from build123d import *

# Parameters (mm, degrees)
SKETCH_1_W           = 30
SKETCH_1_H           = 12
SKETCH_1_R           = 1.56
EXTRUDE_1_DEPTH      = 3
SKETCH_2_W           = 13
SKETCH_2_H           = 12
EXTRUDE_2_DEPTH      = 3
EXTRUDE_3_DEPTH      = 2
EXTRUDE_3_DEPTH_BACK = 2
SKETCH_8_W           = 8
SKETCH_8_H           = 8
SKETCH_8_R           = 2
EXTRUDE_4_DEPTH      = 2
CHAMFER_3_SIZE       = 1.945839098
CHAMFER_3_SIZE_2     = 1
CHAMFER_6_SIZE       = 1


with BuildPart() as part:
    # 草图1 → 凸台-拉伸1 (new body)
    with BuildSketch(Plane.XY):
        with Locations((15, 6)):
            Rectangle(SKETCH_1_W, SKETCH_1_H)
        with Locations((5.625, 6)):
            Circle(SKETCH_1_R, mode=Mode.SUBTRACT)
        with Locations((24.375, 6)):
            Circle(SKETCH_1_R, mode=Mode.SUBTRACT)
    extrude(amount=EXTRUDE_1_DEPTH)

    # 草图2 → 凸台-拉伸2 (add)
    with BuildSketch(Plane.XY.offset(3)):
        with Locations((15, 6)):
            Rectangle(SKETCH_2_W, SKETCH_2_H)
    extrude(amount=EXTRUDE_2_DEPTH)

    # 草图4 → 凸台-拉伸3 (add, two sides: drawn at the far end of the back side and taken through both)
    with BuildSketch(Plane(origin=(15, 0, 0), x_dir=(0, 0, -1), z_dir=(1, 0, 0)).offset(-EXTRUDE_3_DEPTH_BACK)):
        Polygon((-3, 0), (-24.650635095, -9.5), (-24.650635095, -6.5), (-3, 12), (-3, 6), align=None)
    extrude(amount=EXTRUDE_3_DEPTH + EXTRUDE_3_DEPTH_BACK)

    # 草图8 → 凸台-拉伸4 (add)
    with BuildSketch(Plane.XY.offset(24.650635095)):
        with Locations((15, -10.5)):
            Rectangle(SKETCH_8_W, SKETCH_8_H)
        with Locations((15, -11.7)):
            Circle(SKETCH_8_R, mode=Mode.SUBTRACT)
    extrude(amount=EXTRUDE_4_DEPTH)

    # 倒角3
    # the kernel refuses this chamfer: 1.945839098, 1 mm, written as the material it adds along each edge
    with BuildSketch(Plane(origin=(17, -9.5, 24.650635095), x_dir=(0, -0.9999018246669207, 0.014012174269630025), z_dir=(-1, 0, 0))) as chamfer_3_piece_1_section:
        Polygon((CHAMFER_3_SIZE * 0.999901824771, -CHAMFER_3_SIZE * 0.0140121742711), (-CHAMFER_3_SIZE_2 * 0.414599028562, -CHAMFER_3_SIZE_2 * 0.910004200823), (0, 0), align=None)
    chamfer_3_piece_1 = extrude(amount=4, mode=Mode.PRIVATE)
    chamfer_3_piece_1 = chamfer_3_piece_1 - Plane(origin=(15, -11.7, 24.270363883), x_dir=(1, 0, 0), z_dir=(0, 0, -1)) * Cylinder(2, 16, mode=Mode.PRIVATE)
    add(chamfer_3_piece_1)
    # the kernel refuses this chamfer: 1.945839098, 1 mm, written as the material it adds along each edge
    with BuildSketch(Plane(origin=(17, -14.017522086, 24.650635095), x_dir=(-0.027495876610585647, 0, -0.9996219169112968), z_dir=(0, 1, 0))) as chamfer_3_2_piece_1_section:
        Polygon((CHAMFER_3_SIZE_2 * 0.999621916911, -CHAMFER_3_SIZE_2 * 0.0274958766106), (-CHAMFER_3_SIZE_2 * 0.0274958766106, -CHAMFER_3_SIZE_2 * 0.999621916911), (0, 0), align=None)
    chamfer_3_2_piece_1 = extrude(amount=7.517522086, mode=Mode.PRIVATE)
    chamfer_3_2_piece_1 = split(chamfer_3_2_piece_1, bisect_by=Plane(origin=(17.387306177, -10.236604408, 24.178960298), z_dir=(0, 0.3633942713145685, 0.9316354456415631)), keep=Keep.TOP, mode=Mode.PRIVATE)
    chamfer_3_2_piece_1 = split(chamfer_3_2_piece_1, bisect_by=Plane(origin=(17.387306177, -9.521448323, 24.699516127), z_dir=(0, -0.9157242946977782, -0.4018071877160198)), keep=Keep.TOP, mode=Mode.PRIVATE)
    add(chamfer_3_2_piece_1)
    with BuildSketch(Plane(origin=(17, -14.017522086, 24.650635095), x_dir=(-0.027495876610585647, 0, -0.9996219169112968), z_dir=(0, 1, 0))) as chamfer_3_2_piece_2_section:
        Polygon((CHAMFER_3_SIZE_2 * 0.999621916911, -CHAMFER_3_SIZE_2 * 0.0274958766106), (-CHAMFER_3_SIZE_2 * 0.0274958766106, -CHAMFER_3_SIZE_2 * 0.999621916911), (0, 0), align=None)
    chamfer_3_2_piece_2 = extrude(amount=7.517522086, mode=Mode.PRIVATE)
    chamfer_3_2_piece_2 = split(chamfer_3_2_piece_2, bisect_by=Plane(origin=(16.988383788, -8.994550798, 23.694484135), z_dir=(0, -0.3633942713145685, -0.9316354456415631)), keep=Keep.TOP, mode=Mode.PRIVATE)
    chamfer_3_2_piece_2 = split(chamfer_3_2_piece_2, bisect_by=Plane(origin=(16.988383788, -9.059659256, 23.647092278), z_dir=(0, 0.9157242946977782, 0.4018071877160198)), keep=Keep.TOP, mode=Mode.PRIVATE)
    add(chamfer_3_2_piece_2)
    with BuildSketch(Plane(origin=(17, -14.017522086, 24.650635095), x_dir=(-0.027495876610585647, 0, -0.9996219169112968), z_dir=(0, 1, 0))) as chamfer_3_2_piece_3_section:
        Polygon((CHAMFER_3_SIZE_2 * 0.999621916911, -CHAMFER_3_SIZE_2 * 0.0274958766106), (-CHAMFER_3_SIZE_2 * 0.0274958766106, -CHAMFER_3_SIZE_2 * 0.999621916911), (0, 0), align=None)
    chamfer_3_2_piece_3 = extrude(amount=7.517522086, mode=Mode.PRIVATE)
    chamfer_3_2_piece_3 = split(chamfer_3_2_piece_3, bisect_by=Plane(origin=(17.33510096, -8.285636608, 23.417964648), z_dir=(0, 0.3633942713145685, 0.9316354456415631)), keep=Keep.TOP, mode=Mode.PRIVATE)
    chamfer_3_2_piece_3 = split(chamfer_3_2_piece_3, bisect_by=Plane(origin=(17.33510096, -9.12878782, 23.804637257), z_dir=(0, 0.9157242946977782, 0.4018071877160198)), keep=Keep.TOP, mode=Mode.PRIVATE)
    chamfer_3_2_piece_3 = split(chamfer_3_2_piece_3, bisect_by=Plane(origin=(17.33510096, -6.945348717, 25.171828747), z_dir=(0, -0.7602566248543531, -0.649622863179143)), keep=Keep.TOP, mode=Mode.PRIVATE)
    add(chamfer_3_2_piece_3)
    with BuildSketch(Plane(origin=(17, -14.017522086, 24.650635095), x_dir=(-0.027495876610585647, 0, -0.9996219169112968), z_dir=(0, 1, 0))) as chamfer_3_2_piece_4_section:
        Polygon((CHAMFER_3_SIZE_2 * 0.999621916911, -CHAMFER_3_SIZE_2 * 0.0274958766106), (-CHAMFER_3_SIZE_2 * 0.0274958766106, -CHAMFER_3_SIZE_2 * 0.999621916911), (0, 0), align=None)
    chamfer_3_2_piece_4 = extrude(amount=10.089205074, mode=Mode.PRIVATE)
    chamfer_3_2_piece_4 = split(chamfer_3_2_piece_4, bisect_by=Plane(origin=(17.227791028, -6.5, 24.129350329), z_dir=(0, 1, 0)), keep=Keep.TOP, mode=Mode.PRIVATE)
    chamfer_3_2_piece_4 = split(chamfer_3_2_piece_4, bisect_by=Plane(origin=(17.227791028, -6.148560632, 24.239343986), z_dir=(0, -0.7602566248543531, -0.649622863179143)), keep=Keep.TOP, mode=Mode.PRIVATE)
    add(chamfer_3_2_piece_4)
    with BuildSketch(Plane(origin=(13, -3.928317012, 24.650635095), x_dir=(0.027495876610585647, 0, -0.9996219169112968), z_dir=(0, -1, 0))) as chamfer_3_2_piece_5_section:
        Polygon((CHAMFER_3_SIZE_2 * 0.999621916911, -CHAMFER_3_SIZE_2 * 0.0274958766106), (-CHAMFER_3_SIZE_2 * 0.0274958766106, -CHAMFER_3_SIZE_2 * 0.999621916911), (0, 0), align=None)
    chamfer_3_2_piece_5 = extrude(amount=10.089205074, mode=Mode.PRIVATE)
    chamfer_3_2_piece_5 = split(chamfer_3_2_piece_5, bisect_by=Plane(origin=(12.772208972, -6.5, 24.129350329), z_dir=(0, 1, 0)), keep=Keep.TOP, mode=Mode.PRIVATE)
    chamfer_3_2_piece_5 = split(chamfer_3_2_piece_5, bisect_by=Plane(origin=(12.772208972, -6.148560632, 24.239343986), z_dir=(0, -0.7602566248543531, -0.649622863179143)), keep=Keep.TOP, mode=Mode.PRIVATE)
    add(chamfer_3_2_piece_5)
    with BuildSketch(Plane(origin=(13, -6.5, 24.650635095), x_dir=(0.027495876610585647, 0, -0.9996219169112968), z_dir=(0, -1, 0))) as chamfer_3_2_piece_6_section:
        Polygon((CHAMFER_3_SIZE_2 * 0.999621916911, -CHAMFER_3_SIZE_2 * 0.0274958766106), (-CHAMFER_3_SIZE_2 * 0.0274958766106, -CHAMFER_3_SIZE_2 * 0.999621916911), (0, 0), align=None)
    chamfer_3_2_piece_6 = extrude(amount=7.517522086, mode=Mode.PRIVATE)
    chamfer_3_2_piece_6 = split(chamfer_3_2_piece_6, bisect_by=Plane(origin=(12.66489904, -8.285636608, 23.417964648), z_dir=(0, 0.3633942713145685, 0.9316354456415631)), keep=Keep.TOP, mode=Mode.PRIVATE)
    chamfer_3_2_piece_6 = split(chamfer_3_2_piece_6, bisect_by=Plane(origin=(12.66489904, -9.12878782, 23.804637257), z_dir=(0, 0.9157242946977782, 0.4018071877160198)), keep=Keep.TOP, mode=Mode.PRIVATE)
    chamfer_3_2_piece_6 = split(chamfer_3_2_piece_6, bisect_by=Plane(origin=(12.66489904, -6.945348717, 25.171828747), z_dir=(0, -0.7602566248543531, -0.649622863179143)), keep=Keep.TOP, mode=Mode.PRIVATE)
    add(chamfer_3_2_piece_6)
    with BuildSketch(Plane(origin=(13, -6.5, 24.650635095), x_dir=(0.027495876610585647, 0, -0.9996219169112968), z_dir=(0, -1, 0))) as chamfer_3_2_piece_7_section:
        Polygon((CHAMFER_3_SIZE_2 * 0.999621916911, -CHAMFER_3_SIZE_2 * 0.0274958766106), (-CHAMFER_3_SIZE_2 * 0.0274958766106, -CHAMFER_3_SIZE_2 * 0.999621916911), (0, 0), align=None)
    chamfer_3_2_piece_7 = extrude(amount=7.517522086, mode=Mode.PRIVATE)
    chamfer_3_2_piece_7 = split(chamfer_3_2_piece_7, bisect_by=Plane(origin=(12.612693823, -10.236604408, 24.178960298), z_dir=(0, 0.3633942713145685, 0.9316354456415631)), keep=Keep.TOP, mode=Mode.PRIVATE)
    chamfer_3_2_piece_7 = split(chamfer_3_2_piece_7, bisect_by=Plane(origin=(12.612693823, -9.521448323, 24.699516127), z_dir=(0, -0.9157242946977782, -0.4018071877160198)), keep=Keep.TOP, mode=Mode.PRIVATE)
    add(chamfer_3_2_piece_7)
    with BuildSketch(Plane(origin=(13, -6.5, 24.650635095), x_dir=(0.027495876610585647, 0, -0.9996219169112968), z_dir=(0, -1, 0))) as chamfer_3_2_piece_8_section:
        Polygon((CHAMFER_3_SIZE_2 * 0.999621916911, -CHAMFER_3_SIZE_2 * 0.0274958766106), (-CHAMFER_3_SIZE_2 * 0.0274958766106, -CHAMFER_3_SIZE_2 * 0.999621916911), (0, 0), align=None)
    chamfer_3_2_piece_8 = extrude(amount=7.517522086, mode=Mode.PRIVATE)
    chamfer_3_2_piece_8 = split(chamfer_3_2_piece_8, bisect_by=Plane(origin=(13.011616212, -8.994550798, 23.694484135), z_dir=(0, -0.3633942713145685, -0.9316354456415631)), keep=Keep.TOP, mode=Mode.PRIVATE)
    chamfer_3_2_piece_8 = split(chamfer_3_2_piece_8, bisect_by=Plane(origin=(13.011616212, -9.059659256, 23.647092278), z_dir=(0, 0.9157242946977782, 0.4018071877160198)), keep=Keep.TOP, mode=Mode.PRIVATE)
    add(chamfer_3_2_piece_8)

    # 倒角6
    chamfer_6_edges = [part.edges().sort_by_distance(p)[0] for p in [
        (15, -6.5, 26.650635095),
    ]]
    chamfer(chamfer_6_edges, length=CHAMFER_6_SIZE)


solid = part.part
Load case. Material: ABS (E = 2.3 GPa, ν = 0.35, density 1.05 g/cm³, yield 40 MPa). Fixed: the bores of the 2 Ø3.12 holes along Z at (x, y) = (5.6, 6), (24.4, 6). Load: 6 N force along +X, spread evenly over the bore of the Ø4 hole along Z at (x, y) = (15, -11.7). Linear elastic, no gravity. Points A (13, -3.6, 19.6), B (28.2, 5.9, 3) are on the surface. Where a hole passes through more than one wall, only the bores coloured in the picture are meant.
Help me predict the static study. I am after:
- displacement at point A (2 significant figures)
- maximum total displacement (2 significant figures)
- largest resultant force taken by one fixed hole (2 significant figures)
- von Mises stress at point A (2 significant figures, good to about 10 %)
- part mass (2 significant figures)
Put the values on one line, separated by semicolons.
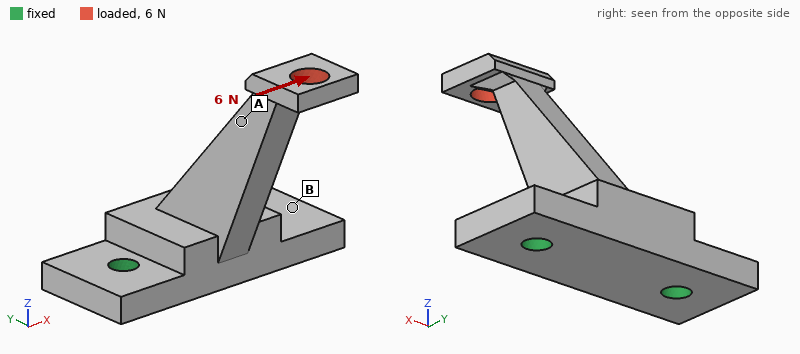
0.18 mm; 0.51 mm; 12 N; 5.0 MPa; 2.2 g
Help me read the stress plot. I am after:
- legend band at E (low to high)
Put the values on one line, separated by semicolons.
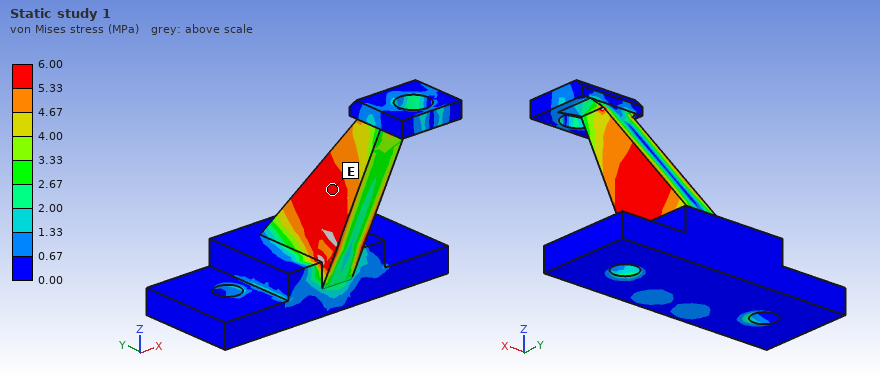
5.33 to 6.00 MPa
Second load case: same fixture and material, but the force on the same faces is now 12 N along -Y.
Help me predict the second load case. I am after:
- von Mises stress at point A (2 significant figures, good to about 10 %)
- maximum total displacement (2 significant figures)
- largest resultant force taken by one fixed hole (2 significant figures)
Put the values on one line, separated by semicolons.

3.6 MPa; 0.49 mm; 6.3 N
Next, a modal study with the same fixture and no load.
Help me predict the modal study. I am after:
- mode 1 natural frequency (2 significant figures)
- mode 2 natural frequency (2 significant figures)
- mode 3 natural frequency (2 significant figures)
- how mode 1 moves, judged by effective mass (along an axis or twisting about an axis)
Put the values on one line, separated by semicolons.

1500 Hz; 1800 Hz; 5500 Hz; along X
